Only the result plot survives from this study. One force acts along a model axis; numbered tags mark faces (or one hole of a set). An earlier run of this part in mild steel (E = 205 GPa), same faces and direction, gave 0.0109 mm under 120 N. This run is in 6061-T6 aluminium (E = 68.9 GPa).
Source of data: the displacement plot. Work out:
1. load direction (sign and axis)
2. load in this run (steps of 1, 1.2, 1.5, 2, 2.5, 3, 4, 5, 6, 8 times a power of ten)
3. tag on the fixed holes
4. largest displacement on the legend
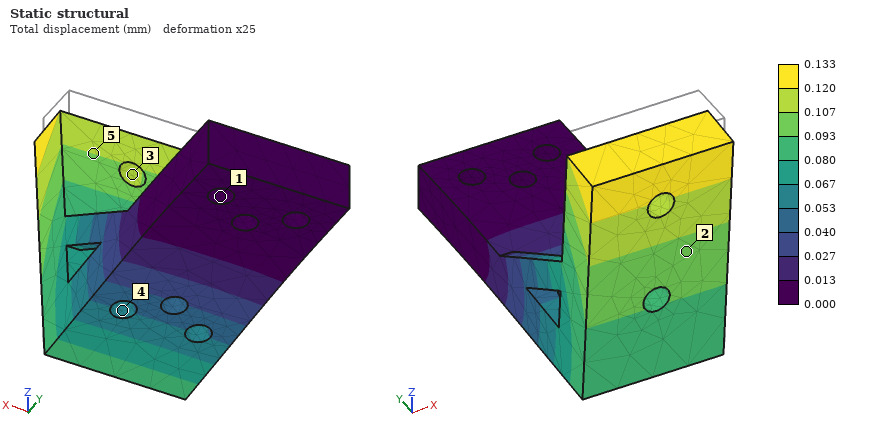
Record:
-Z
500 N
1
0.133 mm
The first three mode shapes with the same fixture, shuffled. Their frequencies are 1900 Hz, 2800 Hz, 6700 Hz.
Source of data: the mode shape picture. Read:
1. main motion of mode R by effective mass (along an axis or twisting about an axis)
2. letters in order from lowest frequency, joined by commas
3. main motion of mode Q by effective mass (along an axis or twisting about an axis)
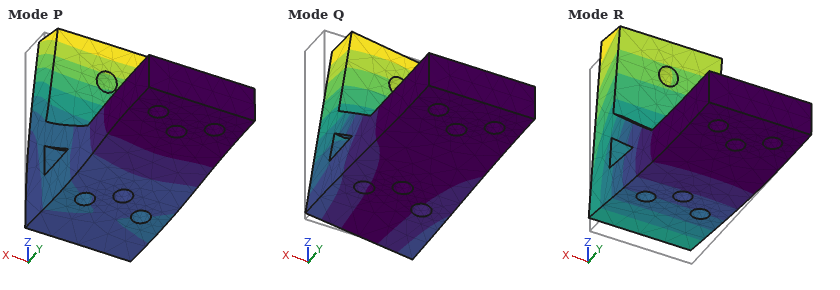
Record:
along Z
R, Q, P
along X
